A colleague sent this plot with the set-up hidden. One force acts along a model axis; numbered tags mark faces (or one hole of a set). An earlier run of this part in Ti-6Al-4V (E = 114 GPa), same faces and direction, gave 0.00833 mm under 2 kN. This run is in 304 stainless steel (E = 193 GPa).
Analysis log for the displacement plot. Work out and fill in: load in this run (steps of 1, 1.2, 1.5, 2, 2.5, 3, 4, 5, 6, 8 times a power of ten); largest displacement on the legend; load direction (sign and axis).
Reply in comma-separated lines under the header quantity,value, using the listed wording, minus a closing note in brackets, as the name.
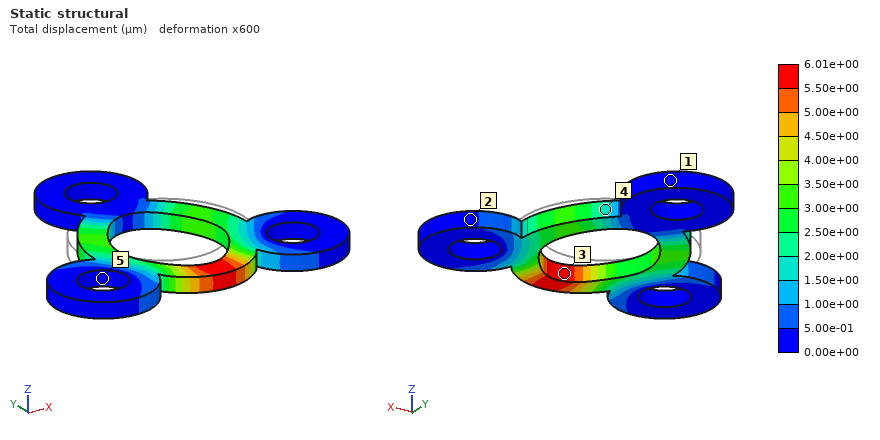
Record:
quantity,value
load in this run,2.5 kN
largest displacement on the legend,6.01e+00 µm
load direction,-Y
